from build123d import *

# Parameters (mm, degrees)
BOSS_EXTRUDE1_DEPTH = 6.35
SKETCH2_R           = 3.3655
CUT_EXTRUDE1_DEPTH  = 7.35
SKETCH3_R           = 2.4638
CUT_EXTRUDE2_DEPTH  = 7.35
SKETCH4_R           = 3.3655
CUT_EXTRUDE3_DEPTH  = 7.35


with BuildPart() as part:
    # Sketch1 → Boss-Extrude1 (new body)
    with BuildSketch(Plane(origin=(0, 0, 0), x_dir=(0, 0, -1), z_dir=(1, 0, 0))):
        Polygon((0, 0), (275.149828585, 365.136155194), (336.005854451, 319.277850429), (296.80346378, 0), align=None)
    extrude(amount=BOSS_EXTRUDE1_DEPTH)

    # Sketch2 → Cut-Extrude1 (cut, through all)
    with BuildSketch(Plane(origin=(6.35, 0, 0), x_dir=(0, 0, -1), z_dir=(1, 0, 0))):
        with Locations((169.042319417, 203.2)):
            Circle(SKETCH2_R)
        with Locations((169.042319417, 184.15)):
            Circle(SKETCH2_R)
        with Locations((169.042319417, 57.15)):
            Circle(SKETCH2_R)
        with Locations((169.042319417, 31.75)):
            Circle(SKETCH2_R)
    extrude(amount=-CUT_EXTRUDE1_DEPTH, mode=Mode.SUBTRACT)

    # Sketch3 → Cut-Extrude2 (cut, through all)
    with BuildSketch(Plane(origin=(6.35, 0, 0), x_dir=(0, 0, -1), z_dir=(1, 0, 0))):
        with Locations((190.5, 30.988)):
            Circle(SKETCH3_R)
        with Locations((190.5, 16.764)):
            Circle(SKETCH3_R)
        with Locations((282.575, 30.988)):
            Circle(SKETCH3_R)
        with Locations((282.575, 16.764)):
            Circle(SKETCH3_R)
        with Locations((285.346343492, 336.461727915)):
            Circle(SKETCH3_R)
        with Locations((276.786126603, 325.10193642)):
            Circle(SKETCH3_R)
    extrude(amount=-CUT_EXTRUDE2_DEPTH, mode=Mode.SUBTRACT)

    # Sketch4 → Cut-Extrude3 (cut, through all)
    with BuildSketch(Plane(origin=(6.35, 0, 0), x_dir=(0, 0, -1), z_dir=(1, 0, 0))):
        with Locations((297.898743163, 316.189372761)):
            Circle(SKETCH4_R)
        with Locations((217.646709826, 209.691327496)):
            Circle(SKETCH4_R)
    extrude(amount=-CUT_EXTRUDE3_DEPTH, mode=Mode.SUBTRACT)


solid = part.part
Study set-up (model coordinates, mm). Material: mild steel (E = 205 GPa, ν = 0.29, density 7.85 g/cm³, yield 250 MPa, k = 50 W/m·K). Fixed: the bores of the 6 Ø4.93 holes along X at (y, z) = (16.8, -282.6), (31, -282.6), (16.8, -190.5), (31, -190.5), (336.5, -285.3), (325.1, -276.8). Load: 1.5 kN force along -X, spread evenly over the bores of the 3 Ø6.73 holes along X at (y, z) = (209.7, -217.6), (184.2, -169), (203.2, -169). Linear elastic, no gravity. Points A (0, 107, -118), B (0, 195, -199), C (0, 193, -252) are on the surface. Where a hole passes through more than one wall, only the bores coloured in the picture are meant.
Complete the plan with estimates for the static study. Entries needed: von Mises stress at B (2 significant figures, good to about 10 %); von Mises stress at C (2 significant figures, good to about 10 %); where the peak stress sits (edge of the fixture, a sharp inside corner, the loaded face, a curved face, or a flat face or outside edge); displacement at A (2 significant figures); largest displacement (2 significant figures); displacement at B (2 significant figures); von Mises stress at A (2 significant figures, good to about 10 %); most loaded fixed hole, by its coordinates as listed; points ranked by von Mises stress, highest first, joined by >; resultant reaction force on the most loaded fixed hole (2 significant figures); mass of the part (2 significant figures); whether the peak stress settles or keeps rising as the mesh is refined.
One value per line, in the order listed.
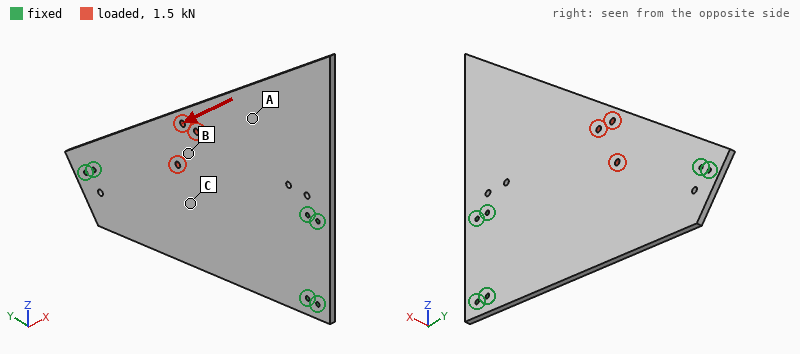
63 MPa
45 MPa
edge of the fixture
0.51 mm
0.98 mm
0.67 mm
16 MPa
(31, -190.5)
B > C > A
3.0 kN
3.2 kg
keeps rising
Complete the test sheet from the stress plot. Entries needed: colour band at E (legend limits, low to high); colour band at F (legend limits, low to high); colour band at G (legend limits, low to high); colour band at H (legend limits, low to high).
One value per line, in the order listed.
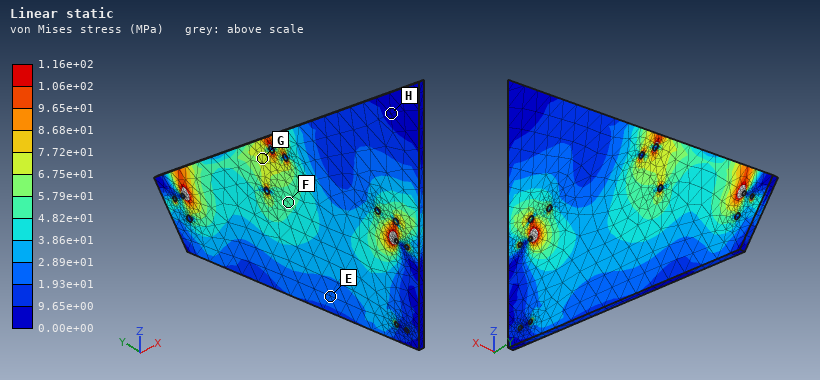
1.93e+01 to 2.89e+01 MPa
4.82e+01 to 5.79e+01 MPa
6.75e+01 to 7.72e+01 MPa
0.00e+00 to 9.65e+00 MPa
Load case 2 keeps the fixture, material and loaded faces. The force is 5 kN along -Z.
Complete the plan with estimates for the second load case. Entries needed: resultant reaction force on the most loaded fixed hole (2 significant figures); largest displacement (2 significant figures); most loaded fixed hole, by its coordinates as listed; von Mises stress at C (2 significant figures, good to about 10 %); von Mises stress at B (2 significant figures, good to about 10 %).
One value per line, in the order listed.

2.4 kN
12 µm
(325.1, -276.8)
4.0 MPa
5.1 MPa
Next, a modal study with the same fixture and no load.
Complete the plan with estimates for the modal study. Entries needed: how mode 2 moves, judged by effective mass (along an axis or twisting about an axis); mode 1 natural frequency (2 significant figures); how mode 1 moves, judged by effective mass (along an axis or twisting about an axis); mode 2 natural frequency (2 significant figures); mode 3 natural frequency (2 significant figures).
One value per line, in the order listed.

along X
210 Hz
along X
290 Hz
440 Hz
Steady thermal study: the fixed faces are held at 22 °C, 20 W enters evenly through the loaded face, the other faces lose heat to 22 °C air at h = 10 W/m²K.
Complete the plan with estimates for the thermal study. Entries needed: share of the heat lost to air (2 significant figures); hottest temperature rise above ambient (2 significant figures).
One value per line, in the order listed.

61 %
37 K
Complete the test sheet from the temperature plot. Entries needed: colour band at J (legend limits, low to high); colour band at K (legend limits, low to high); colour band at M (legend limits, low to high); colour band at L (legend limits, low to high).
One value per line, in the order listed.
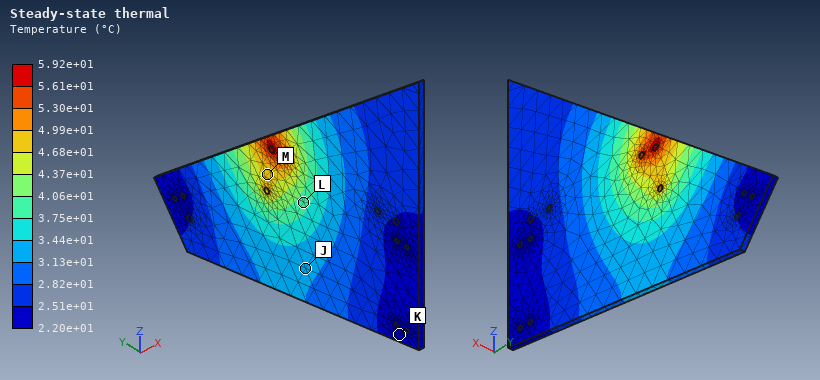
3.13e+01 to 3.44e+01 °C
2.20e+01 to 2.51e+01 °C
4.68e+01 to 4.99e+01 °C
3.75e+01 to 4.06e+01 °C
